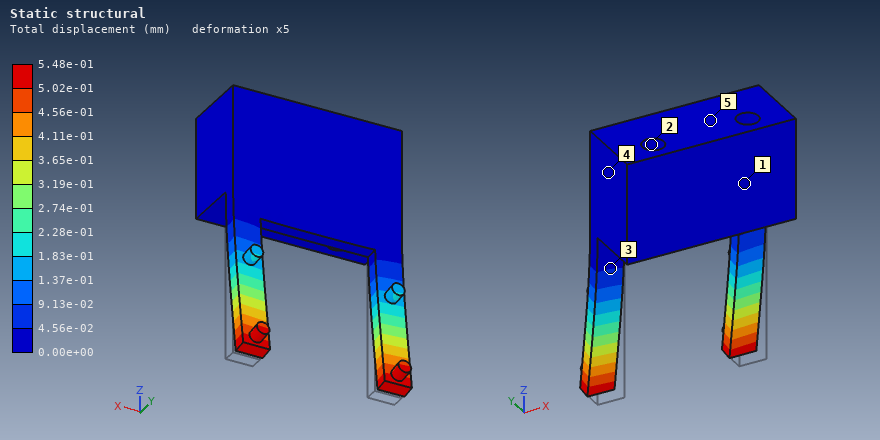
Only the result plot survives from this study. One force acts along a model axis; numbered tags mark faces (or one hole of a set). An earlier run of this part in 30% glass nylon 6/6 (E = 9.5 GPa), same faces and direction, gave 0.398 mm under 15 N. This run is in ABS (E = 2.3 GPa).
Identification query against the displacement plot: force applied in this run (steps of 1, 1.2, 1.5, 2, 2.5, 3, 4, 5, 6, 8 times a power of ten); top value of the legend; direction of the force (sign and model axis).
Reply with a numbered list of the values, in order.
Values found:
1. 5 N
2. 5.48e-01 mm
3. +Y
